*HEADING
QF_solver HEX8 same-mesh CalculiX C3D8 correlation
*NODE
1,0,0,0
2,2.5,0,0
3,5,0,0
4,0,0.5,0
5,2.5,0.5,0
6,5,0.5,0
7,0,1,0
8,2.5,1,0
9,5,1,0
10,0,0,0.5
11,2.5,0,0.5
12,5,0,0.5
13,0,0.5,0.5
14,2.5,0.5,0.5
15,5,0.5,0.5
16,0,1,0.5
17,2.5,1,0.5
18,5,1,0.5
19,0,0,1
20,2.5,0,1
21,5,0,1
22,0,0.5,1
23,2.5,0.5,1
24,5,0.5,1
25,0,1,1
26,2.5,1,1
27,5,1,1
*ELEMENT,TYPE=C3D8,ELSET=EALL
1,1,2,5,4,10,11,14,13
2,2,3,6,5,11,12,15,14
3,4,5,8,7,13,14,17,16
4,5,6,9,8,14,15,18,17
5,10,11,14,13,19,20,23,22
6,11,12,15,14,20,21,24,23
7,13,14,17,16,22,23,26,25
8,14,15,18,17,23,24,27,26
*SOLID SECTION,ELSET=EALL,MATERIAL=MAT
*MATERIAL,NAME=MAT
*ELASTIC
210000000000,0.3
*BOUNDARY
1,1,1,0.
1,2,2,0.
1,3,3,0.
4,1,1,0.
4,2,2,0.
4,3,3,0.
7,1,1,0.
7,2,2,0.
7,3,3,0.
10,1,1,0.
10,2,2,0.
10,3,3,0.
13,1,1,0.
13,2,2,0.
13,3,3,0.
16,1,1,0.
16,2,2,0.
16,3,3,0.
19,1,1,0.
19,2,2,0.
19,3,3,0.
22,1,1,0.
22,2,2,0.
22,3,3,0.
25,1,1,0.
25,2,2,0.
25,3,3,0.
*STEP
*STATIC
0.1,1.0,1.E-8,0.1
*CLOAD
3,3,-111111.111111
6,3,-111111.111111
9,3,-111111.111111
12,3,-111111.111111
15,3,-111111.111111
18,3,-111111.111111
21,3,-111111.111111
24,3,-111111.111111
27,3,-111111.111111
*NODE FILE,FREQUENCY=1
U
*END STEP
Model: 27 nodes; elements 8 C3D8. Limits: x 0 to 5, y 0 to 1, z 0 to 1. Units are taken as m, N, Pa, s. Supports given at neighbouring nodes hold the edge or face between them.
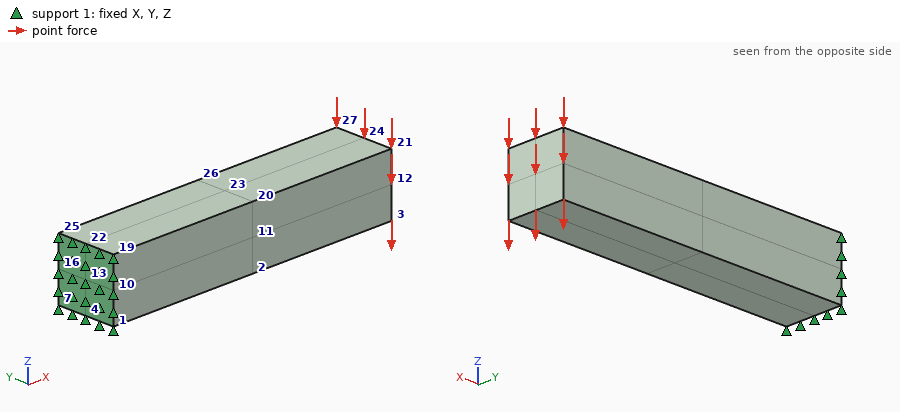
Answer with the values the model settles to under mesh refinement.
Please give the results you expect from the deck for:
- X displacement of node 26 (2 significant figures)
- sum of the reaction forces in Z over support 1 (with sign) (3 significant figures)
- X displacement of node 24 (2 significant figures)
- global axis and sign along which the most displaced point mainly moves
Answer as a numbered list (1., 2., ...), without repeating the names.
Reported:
1. 2.6e-04 m
2. 1.00e+06 N
3. 3.5e-04 m
4. -Z
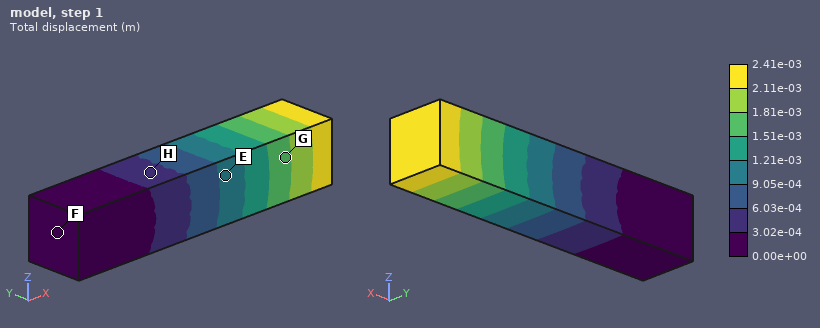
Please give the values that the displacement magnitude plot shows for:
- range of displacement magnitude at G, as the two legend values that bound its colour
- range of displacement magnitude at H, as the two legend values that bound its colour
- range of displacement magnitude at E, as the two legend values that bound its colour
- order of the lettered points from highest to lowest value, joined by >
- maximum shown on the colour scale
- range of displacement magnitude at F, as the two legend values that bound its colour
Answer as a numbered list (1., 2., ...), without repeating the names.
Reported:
1. 1.51e-03 to 1.81e-03 m
2. 3.02e-04 to 6.03e-04 m
3. 9.05e-04 to 1.21e-03 m
4. G > E > H > F
5. 2.41e-03 m
6. 0.00e+00 to 3.02e-04 m
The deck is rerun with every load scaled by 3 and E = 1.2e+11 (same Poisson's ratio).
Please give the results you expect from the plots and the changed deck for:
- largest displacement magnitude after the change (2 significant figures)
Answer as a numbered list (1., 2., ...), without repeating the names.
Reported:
1. 0.013 m
